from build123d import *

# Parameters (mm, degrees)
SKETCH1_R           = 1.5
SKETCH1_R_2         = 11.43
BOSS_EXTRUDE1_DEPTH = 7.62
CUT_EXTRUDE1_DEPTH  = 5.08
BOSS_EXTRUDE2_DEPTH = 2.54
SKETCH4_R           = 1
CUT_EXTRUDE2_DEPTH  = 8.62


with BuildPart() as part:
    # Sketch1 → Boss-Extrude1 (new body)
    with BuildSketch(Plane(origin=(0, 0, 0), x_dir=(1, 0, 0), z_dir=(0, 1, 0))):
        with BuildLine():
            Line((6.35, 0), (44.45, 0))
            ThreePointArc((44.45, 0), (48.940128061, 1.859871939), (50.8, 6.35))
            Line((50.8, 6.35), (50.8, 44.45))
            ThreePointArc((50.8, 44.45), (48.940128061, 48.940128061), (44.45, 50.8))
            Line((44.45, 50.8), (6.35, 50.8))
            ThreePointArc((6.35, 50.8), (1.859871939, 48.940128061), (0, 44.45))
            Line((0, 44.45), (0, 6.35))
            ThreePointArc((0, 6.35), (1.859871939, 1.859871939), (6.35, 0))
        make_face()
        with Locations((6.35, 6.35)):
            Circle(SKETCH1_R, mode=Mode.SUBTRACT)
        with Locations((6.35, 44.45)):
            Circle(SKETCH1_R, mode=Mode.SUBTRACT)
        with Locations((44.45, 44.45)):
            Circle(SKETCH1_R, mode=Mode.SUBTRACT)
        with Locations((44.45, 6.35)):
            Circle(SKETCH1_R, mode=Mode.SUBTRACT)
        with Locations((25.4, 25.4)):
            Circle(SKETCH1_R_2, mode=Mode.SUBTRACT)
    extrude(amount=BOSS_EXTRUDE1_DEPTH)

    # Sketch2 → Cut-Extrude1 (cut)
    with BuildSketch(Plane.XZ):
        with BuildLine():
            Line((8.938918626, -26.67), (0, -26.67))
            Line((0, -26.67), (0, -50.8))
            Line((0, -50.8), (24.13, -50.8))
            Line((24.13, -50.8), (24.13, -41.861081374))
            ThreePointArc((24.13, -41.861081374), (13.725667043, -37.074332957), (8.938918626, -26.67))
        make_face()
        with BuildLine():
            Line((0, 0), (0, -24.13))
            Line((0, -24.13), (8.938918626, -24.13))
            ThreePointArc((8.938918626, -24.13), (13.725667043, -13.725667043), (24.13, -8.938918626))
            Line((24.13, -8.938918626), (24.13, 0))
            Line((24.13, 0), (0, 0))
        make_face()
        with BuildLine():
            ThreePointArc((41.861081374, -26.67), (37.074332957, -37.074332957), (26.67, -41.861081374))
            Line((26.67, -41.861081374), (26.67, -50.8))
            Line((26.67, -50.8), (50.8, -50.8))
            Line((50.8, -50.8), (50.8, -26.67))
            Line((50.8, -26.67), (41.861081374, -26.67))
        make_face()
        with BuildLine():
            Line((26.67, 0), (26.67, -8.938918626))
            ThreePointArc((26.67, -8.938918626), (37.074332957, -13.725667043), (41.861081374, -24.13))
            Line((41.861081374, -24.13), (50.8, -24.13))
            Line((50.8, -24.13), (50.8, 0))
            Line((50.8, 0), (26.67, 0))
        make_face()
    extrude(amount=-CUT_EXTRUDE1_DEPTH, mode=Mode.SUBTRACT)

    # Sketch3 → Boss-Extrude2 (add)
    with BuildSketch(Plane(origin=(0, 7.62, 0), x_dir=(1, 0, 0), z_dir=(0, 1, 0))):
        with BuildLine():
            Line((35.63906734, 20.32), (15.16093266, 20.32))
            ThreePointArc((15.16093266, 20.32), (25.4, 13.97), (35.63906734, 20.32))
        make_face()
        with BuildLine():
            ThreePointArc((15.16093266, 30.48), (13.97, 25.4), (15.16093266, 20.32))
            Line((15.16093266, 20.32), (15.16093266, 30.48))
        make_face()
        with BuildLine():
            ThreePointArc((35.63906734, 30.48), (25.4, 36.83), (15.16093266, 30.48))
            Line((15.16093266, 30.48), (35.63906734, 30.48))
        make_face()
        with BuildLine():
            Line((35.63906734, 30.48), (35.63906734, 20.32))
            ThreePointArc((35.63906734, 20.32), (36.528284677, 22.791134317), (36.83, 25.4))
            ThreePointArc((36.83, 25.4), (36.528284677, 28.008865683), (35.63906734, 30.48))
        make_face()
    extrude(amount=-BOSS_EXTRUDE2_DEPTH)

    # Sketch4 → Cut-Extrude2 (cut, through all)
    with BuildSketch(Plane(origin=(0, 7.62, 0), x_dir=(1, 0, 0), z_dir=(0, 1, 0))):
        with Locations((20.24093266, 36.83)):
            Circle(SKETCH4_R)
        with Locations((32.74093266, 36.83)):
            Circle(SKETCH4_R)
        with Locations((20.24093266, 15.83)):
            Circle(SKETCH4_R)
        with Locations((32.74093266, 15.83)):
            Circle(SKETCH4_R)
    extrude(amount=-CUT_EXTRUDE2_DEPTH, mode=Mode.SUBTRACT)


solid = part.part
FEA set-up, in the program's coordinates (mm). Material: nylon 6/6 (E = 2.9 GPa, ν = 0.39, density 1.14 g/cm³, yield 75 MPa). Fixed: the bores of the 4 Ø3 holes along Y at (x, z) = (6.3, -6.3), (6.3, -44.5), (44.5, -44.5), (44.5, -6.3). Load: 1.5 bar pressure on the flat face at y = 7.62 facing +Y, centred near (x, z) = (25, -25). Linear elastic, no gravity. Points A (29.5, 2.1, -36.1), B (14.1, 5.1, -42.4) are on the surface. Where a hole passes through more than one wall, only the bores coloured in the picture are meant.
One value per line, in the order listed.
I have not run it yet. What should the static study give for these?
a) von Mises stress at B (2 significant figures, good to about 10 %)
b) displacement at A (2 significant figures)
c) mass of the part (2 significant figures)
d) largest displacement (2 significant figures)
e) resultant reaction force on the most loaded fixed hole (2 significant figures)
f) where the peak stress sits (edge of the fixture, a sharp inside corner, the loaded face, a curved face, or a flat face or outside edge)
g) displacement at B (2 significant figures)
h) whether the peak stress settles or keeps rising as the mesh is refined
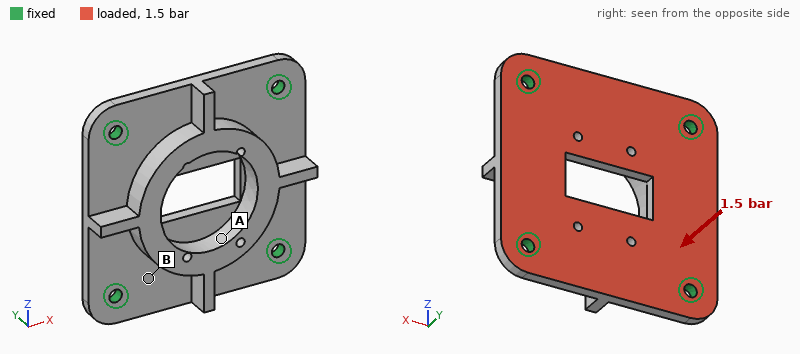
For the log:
5.1 MPa
0.15 mm
9.7 g
0.18 mm
90 N
edge of the fixture
0.092 mm
keeps rising
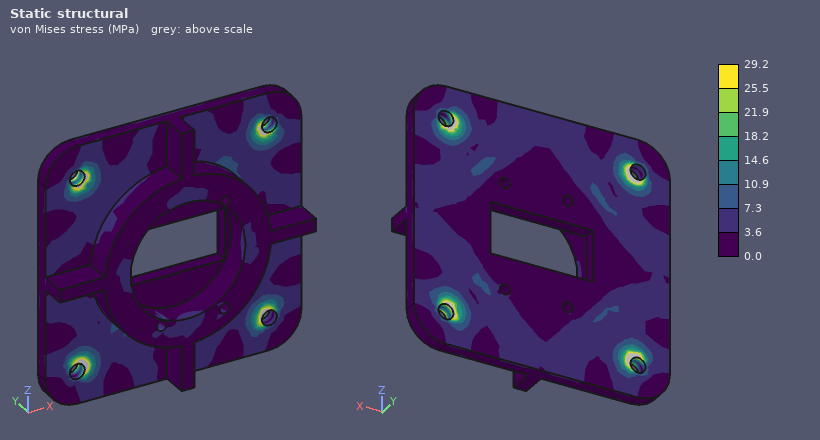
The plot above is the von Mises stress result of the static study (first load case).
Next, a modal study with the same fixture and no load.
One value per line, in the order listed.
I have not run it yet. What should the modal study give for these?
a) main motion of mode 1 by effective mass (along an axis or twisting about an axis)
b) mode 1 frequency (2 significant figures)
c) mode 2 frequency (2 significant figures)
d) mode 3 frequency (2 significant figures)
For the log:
along Y
2400 Hz
3100 Hz
3100 Hz
